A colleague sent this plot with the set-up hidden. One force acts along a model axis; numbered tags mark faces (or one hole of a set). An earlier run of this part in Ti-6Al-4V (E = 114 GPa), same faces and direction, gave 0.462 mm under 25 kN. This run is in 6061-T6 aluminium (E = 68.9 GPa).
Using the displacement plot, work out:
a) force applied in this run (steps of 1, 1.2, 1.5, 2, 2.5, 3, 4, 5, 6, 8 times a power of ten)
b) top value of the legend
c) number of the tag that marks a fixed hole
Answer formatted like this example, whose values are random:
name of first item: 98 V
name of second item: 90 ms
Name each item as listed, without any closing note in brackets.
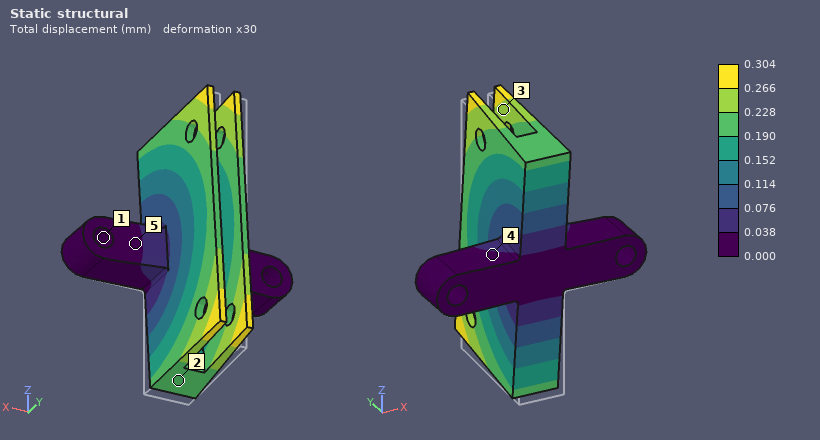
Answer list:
force applied in this run: 10 kN
top value of the legend: 0.304 mm
number of the tag that marks a fixed hole: 1
